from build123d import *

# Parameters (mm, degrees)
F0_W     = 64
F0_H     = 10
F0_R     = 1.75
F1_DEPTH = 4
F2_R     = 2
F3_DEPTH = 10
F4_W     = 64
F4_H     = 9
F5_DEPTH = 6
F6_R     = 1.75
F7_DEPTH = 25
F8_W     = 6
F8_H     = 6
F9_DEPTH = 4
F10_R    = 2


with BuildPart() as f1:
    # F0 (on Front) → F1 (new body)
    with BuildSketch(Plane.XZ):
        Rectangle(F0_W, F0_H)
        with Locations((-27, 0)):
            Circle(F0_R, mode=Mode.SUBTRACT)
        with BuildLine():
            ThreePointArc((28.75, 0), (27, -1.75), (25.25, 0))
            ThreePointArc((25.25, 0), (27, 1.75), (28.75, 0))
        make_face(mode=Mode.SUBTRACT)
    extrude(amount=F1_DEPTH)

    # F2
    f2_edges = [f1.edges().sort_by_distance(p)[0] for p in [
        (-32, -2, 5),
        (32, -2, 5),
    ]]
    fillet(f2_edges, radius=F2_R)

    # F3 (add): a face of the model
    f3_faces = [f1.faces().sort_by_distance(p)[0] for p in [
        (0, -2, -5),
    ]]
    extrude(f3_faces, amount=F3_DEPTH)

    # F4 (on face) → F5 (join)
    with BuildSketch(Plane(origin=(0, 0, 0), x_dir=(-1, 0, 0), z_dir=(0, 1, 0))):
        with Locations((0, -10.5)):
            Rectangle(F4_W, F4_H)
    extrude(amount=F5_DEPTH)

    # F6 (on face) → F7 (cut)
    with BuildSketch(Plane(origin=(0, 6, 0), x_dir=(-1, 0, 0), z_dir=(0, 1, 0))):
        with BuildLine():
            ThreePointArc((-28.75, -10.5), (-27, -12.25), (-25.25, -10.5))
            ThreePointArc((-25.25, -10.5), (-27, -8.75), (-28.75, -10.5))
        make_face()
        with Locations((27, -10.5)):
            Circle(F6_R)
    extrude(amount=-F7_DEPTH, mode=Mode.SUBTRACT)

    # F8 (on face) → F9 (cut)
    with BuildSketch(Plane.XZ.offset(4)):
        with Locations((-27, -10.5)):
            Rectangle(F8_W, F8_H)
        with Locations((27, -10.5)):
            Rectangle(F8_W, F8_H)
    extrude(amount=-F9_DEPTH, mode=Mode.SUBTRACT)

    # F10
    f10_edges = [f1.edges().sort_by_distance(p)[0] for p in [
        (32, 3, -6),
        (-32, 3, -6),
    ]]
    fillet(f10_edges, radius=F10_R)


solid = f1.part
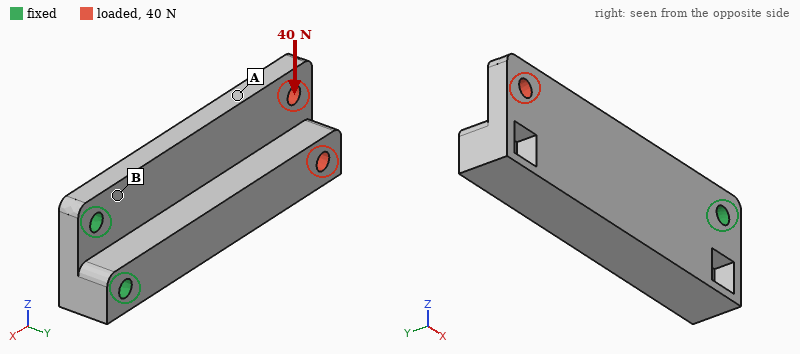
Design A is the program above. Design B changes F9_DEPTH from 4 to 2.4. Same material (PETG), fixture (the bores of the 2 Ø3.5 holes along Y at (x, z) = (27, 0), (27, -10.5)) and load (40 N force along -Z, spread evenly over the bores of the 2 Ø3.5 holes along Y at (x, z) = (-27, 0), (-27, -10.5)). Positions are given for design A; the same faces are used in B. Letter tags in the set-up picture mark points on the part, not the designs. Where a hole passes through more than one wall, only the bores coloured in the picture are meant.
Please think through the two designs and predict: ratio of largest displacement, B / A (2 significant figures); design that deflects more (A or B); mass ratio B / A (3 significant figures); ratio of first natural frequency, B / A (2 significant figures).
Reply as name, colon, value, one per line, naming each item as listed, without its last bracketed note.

ratio of largest displacement, B / A: 0.83
design that deflects more: A
mass ratio B / A: 1.01
ratio of first natural frequency, B / A: 1.1
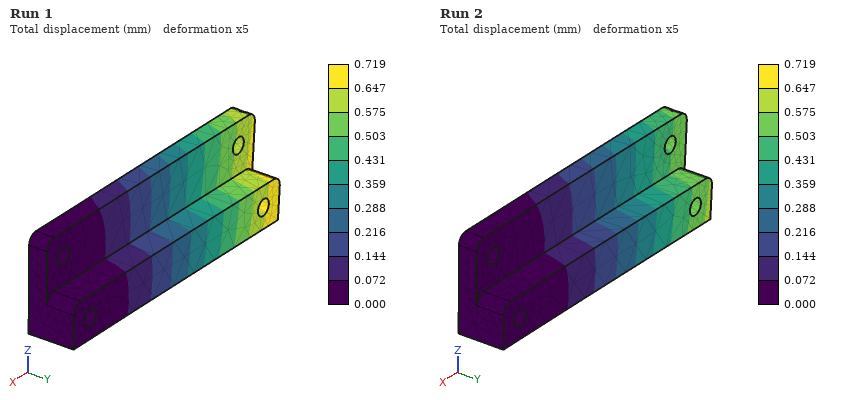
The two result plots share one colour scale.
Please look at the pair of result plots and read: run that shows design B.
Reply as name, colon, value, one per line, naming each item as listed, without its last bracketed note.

run that shows design B: Run 2
